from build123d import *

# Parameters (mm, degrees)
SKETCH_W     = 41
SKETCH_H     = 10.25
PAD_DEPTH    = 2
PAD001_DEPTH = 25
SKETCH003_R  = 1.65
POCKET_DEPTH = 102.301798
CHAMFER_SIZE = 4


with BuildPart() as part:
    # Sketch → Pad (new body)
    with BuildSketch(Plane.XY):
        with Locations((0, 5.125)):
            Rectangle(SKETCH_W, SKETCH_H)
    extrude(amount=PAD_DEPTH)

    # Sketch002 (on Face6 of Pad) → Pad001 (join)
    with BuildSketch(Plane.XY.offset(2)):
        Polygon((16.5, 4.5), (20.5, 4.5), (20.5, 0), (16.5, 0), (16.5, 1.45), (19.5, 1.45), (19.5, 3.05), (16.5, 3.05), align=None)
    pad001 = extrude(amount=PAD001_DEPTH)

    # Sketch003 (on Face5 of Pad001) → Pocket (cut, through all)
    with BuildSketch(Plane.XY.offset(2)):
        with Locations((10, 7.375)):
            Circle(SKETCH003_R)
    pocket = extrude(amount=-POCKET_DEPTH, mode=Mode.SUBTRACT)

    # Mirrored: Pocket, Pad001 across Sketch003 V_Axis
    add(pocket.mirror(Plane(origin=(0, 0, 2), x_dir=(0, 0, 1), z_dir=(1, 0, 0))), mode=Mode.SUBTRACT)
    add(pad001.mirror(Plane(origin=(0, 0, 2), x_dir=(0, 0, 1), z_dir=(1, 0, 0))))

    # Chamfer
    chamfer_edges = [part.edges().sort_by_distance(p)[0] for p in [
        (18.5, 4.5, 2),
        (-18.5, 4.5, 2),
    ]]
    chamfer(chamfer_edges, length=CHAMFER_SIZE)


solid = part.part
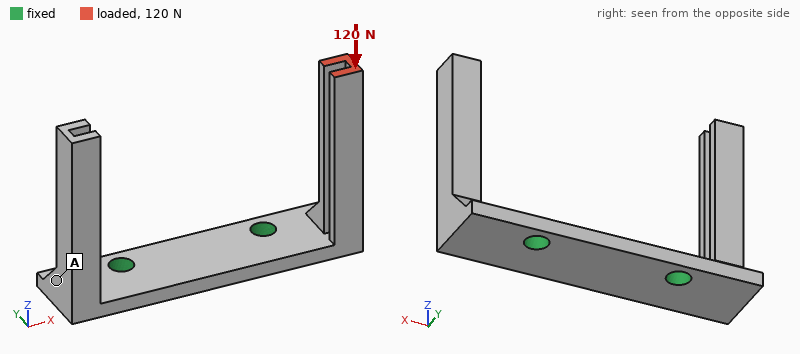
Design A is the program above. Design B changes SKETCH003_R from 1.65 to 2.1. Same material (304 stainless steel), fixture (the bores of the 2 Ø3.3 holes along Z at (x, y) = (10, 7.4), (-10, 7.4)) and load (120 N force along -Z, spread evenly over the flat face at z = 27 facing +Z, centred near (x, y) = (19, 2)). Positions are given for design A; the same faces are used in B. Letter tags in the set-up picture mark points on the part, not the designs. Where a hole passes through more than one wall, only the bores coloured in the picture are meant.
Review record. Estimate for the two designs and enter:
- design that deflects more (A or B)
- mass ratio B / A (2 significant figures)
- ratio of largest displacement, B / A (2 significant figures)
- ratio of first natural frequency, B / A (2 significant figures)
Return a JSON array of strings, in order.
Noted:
["A", "0.99", "0.87", "1.0"]
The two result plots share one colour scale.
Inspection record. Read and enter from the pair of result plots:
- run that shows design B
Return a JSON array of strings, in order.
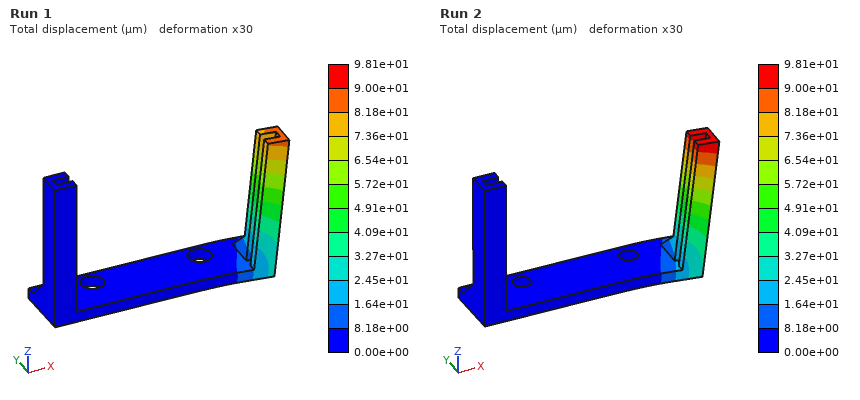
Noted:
["Run 1"]
